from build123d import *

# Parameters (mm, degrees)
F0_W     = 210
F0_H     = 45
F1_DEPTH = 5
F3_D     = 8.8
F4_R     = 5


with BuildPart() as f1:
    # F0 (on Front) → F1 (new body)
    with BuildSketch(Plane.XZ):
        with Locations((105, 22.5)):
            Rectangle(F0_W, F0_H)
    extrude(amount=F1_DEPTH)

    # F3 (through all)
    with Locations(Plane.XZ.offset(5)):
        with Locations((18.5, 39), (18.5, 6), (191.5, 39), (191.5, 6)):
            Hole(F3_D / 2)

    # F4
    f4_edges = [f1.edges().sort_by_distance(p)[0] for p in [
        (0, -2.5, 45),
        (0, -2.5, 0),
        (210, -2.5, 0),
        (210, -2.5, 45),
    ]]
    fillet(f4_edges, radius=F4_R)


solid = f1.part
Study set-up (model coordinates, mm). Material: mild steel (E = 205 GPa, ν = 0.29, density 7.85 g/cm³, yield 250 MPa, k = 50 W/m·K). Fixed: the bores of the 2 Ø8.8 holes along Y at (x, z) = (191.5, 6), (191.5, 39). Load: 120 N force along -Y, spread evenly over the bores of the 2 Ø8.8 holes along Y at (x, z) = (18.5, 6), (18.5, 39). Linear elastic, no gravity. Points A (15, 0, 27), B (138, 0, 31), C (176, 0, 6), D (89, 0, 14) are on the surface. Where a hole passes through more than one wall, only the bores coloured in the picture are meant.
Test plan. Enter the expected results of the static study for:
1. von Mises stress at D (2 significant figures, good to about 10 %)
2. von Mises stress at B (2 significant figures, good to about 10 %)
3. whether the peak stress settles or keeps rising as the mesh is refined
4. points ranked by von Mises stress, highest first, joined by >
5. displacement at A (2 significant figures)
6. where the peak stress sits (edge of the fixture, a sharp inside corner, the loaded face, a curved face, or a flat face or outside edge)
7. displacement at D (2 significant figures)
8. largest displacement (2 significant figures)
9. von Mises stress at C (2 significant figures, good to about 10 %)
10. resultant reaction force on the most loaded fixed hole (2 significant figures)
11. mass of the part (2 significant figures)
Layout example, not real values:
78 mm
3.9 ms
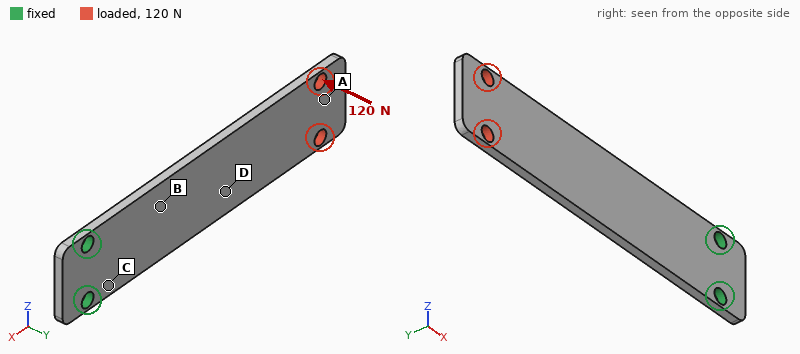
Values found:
45 MPa
76 MPa
keeps rising
C > B > D > A
2.1 mm
edge of the fixture
0.86 mm
2.4 mm
100 MPa
60 N
360 g
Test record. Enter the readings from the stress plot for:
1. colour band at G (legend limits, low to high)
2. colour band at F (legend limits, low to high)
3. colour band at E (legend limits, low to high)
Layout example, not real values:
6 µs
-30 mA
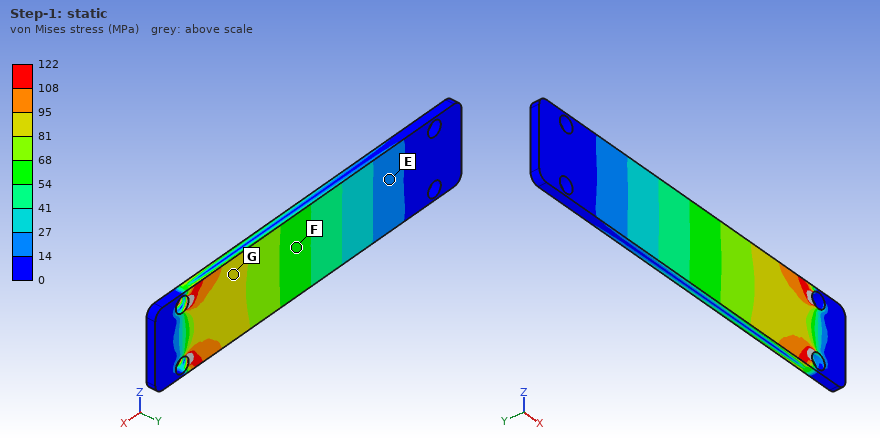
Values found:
81 to 95 MPa
54 to 68 MPa
14 to 27 MPa
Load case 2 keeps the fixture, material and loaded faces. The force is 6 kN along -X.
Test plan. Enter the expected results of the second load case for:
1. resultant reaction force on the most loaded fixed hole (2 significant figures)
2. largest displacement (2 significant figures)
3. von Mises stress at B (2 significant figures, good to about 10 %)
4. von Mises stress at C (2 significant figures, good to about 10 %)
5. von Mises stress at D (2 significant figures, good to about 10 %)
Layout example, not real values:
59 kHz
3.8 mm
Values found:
3.0 kN
25 µm
27 MPa
30 MPa
27 MPa
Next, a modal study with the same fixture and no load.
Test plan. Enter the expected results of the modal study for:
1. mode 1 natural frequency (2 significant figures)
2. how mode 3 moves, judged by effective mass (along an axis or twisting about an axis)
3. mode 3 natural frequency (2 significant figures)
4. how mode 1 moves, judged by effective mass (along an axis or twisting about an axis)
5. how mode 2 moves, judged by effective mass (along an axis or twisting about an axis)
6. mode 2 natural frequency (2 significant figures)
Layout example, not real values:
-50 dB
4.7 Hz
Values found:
120 Hz
twisting about X
990 Hz
along Y
along Y
730 Hz
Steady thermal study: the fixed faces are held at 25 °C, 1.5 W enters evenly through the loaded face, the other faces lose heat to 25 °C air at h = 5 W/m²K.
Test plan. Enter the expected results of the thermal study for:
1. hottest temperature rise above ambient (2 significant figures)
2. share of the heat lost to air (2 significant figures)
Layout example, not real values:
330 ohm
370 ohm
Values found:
16 K
48 %
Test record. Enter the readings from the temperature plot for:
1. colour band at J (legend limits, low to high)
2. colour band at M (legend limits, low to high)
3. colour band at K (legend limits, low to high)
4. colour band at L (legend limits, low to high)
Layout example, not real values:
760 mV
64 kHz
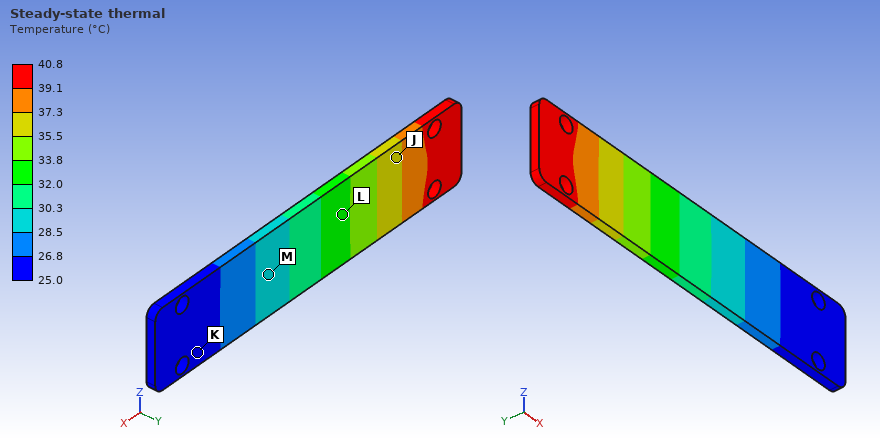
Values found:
35.5 to 37.3 °C
28.5 to 30.3 °C
25.0 to 26.8 °C
32.0 to 33.8 °C
